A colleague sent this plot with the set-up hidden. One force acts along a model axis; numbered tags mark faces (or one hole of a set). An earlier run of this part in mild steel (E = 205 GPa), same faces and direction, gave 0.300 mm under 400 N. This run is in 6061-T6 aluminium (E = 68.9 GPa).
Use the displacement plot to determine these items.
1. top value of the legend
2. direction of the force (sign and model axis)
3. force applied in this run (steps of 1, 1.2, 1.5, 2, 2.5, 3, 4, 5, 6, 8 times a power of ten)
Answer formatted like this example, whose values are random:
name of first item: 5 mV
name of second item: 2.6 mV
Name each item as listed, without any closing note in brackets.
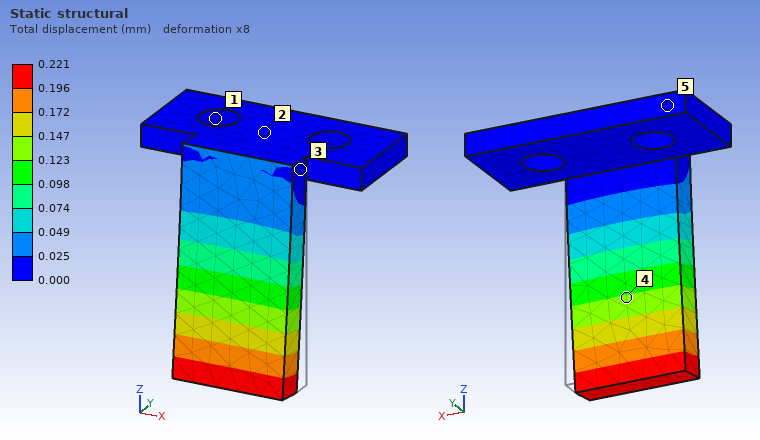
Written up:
top value of the legend: 0.221 mm
direction of the force: -Y
force applied in this run: 100 N
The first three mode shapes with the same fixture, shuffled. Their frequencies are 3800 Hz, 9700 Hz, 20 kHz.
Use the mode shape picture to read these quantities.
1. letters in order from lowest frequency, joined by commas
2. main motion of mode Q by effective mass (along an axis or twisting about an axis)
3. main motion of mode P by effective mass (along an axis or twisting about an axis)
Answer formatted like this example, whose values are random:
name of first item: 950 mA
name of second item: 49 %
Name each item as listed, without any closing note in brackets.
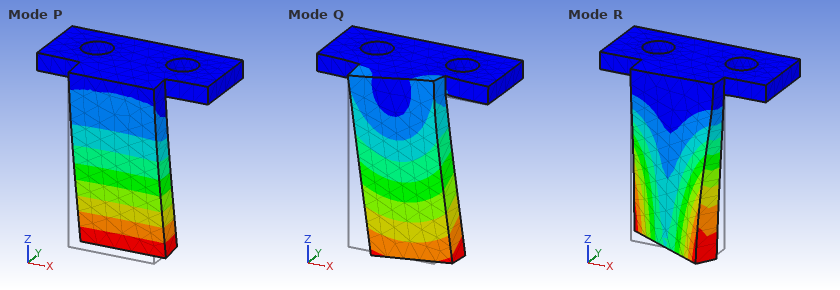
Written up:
letters in order from lowest frequency, joined by commas: P, Q, R
main motion of mode Q by effective mass: along X
main motion of mode P by effective mass: along Y
